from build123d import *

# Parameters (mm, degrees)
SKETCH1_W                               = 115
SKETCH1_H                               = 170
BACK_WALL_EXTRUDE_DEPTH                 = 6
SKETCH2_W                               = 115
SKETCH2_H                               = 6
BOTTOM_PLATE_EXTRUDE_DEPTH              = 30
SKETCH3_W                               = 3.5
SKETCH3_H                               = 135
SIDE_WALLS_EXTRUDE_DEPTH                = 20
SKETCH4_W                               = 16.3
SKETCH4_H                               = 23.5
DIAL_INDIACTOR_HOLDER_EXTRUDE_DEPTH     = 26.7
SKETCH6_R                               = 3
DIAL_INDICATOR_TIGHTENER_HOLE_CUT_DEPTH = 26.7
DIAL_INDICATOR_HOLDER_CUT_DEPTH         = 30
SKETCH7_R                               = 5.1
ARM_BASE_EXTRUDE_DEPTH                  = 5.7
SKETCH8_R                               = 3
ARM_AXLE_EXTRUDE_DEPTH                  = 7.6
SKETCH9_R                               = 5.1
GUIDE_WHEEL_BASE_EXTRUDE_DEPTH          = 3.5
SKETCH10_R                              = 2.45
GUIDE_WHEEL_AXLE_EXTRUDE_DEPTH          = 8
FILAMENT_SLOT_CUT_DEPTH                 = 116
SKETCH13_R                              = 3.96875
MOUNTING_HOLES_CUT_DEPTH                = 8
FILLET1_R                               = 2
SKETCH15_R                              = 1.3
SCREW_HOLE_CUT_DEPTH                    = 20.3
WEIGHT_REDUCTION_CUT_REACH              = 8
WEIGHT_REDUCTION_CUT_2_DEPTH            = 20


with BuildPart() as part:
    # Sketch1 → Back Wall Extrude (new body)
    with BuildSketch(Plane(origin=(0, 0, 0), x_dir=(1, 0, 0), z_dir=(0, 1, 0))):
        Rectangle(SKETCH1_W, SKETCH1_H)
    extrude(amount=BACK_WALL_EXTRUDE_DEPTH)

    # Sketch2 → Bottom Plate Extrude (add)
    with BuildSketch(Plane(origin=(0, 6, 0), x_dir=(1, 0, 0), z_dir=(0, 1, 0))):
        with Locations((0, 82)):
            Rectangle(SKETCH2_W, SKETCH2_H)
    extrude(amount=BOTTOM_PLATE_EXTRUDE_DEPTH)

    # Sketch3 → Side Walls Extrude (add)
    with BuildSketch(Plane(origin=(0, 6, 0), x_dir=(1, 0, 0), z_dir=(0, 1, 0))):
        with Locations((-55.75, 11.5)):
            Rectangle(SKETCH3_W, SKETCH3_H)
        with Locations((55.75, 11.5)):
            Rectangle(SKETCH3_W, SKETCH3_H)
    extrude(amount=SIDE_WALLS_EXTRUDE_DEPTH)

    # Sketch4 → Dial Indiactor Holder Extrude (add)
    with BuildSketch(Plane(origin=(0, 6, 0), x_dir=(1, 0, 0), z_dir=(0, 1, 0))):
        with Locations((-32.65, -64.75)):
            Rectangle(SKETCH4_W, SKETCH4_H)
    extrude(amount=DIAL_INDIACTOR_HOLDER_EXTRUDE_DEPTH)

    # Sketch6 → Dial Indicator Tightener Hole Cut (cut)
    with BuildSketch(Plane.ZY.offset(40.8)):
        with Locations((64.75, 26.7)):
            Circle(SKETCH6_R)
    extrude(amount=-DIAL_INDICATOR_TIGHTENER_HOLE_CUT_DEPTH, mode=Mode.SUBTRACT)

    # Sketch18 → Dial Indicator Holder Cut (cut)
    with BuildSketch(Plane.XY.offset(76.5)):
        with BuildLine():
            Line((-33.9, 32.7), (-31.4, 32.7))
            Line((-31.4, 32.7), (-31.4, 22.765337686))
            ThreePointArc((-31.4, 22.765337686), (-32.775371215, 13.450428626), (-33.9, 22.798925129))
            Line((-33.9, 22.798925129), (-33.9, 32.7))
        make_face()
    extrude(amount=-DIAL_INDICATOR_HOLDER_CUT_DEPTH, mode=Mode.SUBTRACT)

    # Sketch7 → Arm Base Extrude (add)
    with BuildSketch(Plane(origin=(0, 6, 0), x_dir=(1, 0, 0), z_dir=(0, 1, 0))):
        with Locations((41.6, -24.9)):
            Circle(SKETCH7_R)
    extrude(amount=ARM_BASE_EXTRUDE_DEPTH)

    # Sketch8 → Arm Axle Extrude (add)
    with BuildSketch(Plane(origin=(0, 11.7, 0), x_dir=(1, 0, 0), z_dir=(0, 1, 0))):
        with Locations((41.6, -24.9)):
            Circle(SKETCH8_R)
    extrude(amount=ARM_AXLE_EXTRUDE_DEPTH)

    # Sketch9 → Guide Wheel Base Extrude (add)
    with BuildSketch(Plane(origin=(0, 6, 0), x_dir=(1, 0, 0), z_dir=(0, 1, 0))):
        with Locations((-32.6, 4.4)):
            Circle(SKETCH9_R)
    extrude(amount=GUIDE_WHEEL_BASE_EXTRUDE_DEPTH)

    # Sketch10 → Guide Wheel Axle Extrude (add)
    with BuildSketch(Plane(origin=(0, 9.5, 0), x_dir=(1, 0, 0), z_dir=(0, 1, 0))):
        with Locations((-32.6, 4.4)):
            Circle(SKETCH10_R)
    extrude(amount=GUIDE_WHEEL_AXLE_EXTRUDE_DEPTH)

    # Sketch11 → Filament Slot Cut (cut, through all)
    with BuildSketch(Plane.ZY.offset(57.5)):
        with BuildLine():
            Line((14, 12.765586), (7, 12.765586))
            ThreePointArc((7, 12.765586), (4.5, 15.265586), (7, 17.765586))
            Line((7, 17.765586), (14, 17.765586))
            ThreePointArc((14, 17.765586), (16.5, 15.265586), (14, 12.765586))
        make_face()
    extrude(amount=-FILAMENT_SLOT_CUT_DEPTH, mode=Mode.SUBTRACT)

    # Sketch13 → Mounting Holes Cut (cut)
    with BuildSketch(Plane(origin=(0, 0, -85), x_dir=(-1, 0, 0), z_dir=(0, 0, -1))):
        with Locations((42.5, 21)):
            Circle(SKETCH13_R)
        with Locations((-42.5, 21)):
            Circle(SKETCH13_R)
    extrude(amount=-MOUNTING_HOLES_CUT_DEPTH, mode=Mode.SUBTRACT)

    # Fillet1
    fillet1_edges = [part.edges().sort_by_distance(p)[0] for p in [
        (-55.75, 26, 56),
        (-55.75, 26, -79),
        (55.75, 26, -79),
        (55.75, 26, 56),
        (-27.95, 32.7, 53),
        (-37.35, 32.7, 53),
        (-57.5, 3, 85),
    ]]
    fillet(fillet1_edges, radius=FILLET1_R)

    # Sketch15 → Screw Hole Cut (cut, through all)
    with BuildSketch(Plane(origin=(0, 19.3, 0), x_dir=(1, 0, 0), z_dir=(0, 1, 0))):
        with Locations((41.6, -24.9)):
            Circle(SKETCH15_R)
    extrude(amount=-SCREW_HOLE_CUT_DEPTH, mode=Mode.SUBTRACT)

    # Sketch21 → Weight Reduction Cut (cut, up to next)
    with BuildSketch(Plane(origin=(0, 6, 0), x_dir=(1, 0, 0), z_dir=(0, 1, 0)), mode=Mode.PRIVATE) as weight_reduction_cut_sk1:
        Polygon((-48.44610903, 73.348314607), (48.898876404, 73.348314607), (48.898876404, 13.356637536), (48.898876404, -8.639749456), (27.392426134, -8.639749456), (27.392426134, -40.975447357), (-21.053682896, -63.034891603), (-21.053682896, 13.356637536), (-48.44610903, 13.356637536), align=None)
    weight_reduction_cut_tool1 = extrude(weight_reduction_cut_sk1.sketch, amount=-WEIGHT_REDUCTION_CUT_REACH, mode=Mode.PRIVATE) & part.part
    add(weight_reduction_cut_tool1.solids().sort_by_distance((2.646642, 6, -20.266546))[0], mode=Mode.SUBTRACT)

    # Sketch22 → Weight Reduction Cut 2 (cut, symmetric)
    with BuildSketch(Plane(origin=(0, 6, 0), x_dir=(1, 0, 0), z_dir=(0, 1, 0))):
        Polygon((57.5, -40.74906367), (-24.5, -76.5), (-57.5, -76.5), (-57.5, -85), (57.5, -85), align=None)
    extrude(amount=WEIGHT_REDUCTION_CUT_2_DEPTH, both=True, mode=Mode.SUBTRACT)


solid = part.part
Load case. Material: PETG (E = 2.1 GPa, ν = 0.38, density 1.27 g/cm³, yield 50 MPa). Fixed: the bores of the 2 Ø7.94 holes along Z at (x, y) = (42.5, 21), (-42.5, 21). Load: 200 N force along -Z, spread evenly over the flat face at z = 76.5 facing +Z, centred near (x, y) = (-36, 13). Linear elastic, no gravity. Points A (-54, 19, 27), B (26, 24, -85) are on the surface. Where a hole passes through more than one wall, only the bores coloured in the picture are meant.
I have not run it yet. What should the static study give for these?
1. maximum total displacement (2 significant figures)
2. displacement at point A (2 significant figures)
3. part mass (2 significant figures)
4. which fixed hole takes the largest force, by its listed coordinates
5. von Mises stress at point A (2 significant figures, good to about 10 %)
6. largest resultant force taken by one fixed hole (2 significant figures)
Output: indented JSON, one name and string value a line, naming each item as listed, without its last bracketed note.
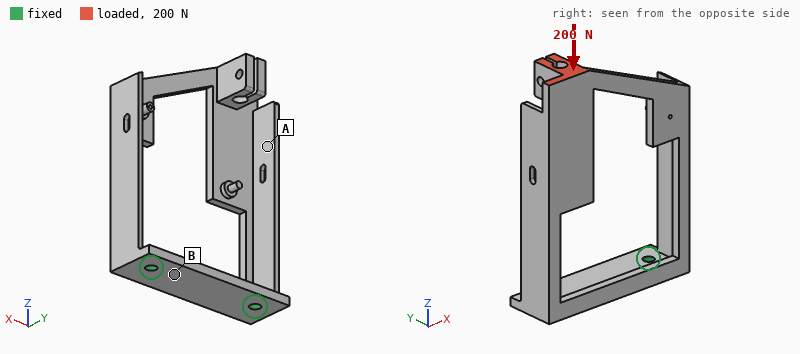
{
  "maximum total displacement": "1.4 mm",
  "displacement at point A": "0.38 mm",
  "part mass": "120 g",
  "which fixed hole takes the largest force, by its listed coordinates": "(-42.5, 21)",
  "von Mises stress at point A": "1.6 MPa",
  "largest resultant force taken by one fixed hole": "170 N"
}
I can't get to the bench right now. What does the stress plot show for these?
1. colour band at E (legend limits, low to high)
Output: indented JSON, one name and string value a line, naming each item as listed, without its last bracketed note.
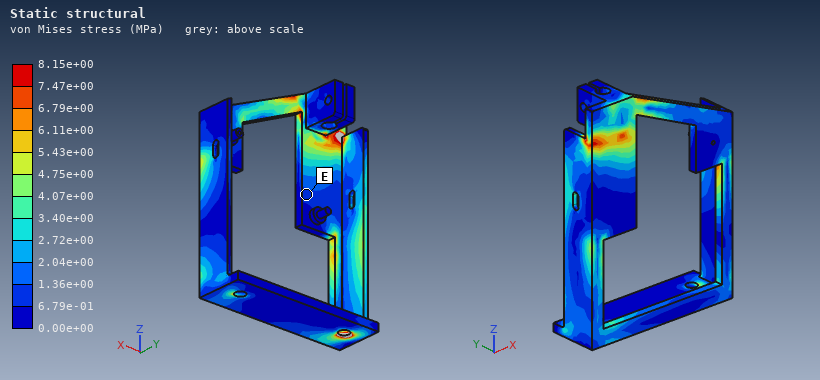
{
  "colour band at E": "6.79e-01 to 1.36e+00 MPa"
}
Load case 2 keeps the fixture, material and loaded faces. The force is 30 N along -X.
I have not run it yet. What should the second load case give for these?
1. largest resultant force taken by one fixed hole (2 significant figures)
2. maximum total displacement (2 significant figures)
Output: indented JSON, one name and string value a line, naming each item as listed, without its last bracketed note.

{
  "largest resultant force taken by one fixed hole": "47 N",
  "maximum total displacement": "2.4 mm"
}
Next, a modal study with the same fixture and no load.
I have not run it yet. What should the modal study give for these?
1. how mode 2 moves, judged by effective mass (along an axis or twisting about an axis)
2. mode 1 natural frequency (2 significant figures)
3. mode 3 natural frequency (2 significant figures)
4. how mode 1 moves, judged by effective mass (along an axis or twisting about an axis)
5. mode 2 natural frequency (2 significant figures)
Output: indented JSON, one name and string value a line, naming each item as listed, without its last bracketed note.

{
  "how mode 2 moves, judged by effective mass": "along X",
  "mode 1 natural frequency": "75 Hz",
  "mode 3 natural frequency": "170 Hz",
  "how mode 1 moves, judged by effective mass": "along Y",
  "mode 2 natural frequency": "94 Hz"
}
